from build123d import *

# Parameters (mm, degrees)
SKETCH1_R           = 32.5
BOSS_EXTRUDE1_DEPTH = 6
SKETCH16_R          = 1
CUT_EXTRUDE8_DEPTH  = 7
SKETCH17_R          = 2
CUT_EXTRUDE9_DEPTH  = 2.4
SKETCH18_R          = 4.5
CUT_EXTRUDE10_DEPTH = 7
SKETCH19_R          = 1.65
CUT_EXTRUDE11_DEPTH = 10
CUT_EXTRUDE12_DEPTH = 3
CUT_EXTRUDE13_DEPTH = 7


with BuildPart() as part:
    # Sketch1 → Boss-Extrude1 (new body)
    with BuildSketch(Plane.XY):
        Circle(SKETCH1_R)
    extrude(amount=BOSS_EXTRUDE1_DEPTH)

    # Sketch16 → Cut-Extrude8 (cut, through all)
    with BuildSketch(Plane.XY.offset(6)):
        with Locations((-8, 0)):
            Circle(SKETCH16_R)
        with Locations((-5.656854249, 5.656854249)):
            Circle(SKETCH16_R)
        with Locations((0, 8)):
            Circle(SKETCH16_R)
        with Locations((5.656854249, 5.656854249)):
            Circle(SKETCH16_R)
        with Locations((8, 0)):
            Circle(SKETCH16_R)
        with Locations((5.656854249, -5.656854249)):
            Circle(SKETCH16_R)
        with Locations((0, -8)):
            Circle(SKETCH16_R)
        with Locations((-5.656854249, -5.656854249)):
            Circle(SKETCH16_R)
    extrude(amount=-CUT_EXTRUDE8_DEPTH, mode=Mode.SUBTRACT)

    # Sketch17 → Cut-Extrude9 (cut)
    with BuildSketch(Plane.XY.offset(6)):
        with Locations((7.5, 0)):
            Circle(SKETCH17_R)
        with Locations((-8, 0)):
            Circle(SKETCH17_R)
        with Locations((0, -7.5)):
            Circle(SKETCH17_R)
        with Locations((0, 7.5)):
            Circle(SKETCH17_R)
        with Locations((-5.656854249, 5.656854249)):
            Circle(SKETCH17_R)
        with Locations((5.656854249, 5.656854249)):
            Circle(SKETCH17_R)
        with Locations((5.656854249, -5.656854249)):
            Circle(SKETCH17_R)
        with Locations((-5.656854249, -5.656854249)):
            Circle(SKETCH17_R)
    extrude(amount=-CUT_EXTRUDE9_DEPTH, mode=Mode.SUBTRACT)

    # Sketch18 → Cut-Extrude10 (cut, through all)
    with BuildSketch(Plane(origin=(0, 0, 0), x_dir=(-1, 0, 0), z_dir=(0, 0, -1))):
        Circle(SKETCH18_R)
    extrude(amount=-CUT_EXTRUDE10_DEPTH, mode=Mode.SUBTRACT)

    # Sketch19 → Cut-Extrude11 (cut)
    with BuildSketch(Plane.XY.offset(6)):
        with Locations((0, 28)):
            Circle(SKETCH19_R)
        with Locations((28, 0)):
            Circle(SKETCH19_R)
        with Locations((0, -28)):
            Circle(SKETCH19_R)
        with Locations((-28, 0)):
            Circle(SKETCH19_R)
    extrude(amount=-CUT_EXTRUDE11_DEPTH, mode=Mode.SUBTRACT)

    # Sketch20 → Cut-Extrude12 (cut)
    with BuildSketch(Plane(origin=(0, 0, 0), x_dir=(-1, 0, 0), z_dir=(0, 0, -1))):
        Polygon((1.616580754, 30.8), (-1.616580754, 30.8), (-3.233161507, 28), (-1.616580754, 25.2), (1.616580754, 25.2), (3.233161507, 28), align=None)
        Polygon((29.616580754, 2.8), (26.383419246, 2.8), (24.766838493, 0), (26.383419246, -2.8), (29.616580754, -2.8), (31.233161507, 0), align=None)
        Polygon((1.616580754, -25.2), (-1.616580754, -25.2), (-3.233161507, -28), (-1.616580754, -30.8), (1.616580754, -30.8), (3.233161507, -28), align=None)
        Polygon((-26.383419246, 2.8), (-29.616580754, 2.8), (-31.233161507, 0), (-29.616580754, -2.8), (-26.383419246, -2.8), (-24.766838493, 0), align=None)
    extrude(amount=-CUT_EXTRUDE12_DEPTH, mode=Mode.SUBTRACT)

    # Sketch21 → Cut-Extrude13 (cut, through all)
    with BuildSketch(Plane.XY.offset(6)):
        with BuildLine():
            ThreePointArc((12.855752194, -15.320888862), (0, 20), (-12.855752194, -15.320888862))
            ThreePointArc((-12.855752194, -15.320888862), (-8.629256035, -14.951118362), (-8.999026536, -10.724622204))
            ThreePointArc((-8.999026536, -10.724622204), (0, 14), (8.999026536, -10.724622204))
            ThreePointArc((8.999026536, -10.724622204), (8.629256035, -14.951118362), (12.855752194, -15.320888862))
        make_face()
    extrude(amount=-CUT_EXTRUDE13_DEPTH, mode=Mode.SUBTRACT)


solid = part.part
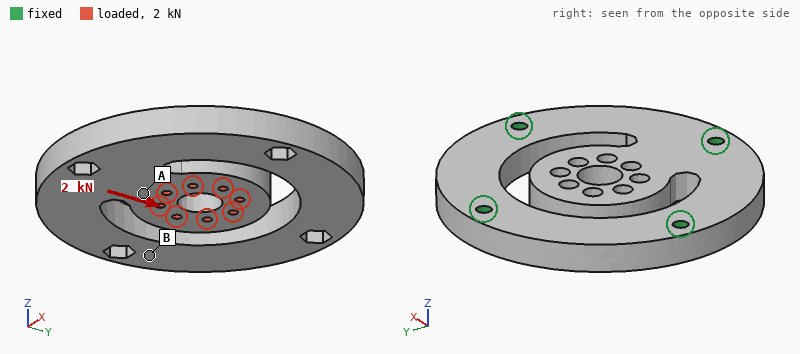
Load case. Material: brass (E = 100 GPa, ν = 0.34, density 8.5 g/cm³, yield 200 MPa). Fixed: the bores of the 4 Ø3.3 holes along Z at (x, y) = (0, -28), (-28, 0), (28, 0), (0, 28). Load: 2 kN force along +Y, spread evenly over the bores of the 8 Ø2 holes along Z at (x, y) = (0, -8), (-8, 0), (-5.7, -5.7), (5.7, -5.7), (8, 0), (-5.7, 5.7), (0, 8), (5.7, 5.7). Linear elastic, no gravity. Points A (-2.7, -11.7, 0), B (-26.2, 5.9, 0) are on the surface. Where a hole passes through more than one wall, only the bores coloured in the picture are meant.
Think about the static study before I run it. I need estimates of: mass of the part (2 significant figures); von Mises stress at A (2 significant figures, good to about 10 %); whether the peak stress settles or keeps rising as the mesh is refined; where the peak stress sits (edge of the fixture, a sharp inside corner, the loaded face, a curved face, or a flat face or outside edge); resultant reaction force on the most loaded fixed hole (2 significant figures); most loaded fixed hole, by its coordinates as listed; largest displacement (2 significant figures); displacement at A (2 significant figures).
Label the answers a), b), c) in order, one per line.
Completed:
a) 130 g
b) 35 MPa
c) keeps rising
d) edge of the fixture
e) 1.4 kN
f) (0, -28)
g) 75 µm
h) 19 µm
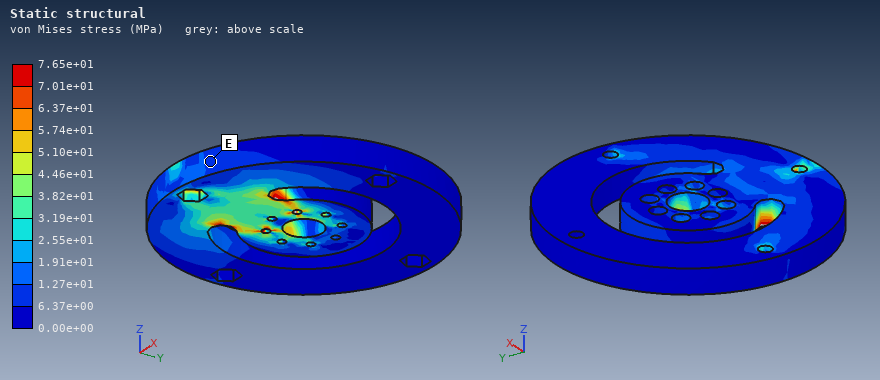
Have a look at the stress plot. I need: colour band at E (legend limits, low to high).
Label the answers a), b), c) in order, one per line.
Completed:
a) 6.37e+00 to 1.27e+01 MPa
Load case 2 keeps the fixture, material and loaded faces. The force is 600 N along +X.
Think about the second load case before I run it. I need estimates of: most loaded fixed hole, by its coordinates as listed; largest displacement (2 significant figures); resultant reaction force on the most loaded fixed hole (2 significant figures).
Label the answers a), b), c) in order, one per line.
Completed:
a) (0, -28)
b) 36 µm
c) 630 N
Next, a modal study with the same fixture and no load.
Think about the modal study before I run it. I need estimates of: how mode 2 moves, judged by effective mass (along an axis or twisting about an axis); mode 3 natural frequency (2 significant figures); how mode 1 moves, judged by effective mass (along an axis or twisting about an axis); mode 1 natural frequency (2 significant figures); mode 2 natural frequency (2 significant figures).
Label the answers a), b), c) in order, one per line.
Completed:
a) along X
b) 5200 Hz
c) along Z
d) 1800 Hz
e) 4500 Hz
